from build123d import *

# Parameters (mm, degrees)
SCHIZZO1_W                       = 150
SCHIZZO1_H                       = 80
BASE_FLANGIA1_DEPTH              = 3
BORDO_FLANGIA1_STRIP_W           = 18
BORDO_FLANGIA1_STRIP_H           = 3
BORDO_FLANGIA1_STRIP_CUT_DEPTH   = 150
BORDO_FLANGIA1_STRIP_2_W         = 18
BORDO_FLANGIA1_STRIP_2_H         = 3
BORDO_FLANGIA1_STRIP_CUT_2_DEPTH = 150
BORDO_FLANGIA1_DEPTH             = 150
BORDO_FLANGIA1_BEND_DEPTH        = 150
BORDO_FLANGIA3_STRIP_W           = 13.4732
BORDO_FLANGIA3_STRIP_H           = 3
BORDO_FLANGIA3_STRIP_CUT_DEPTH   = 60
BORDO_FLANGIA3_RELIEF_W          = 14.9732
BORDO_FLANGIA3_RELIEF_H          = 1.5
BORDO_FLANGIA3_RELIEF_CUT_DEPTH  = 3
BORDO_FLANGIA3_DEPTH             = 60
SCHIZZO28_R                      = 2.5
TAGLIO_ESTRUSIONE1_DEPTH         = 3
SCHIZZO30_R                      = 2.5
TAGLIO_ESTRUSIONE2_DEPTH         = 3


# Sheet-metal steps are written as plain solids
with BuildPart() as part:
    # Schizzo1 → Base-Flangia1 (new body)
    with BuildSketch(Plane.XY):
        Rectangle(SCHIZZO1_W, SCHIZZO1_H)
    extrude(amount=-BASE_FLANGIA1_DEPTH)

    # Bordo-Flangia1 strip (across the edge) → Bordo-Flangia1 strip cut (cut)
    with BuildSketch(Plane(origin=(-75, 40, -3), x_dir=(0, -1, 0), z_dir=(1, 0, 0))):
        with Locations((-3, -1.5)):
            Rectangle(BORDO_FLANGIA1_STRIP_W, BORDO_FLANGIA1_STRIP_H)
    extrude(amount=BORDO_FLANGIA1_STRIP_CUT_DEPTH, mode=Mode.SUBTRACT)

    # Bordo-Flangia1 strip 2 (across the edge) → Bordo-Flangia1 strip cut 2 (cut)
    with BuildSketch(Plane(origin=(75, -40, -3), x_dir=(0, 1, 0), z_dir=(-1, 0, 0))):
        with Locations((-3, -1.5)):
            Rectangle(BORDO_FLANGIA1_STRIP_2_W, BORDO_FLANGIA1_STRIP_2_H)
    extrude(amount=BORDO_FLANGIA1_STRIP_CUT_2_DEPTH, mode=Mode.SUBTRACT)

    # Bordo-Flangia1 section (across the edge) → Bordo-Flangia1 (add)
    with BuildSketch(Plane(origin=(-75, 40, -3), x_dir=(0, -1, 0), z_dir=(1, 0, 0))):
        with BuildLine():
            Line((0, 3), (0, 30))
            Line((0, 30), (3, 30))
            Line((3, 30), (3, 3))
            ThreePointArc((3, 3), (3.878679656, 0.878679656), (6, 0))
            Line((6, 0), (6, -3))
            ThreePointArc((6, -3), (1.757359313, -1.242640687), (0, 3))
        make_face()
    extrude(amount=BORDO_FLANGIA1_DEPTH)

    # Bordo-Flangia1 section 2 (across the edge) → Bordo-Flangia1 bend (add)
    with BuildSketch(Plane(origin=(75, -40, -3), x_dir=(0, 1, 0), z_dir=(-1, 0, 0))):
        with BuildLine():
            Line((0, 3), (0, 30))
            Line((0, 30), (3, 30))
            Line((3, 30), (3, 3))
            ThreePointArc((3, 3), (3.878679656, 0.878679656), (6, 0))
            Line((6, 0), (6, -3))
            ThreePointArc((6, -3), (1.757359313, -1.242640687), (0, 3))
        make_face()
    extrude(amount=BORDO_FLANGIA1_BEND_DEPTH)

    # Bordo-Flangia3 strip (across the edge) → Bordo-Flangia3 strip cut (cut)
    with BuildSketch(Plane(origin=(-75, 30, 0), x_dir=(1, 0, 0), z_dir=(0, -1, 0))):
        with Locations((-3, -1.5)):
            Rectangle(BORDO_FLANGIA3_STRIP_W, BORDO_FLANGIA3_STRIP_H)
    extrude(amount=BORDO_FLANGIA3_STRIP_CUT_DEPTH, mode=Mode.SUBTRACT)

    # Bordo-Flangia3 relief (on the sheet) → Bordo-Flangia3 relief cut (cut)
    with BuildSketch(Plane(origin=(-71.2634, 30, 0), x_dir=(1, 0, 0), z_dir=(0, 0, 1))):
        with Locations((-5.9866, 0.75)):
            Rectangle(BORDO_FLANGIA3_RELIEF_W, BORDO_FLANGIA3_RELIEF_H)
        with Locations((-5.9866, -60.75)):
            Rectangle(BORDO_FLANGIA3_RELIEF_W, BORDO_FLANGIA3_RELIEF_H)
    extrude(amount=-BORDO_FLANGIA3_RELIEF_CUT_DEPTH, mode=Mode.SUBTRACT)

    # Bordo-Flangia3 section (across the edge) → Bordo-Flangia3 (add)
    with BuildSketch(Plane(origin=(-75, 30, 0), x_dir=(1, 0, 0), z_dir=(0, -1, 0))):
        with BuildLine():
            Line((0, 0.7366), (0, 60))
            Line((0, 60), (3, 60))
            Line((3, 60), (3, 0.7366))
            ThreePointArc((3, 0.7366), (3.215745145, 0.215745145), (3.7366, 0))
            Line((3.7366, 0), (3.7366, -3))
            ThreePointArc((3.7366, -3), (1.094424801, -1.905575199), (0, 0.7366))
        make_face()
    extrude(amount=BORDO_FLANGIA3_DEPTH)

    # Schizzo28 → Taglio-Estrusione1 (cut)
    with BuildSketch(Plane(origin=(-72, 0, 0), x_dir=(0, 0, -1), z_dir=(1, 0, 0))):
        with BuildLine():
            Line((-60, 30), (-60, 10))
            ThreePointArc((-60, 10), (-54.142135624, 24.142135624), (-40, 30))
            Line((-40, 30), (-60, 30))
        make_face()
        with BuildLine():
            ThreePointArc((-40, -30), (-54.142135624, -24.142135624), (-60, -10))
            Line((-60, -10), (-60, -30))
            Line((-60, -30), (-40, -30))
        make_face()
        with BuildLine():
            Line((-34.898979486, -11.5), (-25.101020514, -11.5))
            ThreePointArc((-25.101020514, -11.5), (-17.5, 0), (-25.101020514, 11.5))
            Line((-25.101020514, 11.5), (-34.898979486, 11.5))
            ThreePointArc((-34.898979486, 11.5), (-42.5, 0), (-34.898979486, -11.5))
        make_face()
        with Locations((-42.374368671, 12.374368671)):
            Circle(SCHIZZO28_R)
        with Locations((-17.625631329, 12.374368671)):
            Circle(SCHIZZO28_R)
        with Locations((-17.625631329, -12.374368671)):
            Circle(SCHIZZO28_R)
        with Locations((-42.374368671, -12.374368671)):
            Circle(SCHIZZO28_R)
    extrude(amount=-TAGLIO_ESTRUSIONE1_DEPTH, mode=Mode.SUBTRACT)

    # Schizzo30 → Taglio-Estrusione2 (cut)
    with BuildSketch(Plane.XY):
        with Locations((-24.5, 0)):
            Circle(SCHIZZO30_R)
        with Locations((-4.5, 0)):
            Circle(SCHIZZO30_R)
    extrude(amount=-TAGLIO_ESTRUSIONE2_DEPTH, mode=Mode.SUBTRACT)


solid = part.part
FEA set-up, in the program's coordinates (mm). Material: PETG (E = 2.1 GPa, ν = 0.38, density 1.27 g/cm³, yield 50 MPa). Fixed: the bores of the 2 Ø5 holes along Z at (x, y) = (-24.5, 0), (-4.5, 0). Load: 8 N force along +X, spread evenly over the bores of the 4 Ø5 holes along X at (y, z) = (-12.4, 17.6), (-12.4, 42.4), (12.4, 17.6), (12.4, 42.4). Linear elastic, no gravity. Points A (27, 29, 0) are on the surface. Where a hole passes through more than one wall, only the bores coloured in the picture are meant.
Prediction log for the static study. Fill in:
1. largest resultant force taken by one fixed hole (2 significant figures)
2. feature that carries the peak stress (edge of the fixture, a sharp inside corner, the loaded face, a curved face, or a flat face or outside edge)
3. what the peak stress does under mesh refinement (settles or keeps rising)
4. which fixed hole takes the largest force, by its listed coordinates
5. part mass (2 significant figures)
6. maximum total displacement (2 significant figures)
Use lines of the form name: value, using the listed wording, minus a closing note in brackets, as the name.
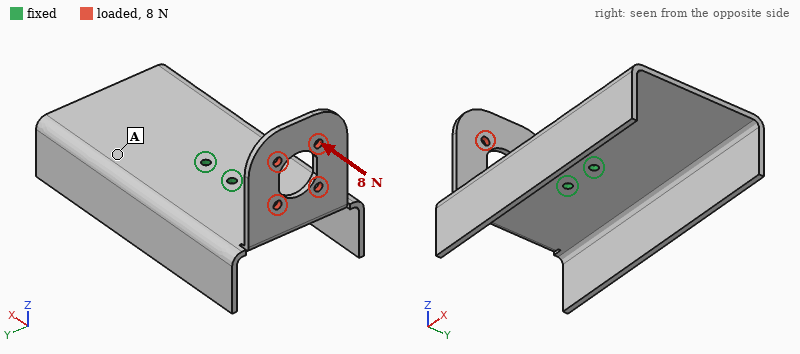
largest resultant force taken by one fixed hole: 9.5 N
feature that carries the peak stress: a sharp inside corner
what the peak stress does under mesh refinement: keeps rising
which fixed hole takes the largest force, by its listed coordinates: (-24.5, 0)
part mass: 88 g
maximum total displacement: 1.9 mm
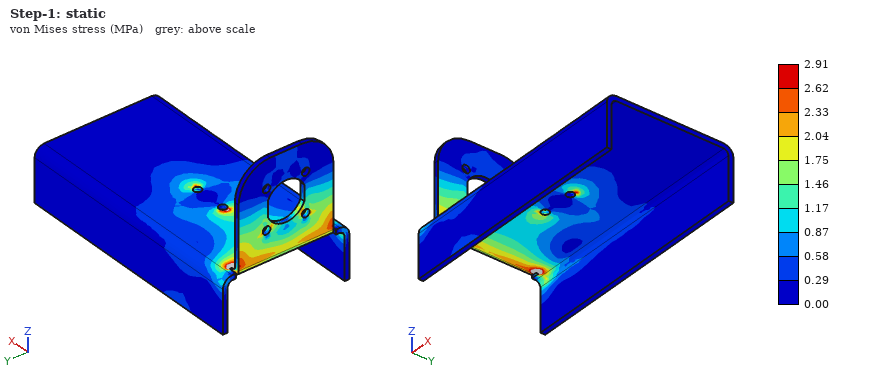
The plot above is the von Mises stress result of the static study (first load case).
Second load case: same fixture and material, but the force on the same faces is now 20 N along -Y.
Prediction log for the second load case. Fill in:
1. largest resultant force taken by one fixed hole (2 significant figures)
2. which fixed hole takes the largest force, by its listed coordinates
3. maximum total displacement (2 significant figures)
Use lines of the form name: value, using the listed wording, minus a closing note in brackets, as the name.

largest resultant force taken by one fixed hole: 60 N
which fixed hole takes the largest force, by its listed coordinates: (-24.5, 0)
maximum total displacement: 2.1 mm
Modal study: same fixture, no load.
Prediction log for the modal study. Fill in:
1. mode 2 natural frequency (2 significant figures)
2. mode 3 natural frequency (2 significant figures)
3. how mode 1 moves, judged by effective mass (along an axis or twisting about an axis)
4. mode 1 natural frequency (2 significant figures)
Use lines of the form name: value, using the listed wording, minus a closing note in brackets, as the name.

mode 2 natural frequency: 110 Hz
mode 3 natural frequency: 120 Hz
how mode 1 moves, judged by effective mass: twisting about Y
mode 1 natural frequency: 88 Hz
